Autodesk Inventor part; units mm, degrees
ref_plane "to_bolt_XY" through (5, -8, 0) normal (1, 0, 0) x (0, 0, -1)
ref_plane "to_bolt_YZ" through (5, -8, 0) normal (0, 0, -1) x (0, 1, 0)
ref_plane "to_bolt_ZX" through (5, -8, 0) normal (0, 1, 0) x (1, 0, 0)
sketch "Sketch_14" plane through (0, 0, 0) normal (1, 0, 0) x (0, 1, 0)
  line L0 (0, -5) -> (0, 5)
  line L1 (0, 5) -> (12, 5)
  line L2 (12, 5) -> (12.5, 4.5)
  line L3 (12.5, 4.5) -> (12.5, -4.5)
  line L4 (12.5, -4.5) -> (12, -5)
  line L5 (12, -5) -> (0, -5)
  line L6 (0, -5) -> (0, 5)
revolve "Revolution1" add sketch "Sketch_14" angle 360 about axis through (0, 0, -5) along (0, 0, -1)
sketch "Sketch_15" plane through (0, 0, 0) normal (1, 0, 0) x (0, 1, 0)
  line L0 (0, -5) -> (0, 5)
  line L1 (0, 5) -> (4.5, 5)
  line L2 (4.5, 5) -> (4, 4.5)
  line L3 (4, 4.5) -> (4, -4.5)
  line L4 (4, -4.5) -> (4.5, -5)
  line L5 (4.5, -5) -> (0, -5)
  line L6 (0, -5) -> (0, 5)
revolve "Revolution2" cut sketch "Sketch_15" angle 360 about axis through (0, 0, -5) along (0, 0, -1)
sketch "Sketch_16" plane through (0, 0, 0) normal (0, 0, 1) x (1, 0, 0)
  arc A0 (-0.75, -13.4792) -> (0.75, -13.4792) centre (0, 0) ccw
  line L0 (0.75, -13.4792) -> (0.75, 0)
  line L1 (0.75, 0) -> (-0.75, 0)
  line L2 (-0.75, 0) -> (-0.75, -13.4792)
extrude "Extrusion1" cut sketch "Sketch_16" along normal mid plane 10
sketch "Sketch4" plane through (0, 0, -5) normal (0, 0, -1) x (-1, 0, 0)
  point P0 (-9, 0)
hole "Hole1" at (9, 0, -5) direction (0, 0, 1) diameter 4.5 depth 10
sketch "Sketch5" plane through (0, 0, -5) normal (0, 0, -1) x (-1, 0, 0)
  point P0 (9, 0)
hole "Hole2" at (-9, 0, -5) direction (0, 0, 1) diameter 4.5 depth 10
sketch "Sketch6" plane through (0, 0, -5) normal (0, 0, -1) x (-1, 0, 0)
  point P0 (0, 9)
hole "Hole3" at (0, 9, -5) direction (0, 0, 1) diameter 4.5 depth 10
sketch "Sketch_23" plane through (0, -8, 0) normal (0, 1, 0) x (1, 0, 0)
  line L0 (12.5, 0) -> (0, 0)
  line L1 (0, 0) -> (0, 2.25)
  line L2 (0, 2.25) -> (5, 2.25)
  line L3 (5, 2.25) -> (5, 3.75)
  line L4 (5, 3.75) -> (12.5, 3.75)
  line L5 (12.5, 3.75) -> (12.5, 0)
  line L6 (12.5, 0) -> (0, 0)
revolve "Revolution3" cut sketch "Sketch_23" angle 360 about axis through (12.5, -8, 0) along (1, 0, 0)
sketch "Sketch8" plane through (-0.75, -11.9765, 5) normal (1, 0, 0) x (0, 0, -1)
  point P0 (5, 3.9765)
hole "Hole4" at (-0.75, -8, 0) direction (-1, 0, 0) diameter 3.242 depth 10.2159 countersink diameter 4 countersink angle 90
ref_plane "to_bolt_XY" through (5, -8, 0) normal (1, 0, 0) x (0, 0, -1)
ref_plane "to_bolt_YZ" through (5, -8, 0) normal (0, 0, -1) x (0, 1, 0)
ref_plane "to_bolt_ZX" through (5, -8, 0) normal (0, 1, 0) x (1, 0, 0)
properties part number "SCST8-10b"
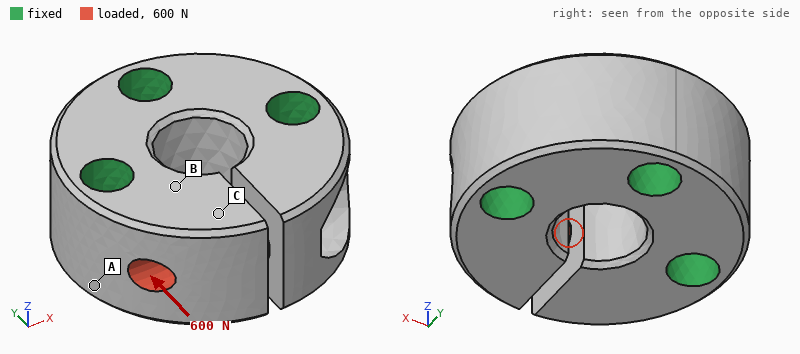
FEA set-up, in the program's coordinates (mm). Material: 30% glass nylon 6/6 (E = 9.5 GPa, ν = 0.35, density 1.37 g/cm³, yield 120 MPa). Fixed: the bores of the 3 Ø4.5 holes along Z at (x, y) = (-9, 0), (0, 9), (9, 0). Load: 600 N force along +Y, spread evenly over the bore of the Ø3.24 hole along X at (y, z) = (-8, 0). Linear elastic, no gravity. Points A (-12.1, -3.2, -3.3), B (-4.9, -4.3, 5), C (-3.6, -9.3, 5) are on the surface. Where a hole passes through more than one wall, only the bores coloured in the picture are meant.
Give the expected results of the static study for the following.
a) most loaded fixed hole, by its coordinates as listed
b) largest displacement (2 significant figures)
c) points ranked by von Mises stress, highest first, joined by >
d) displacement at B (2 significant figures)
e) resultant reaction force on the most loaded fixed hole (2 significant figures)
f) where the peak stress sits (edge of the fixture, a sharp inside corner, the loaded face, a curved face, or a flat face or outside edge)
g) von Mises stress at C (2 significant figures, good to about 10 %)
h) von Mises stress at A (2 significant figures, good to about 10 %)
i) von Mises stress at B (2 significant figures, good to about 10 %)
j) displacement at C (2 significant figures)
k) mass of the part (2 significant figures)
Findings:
(-9, 0)
35 µm
B > A > C
10.0 µm
530 N
the loaded face
2.5 MPa
6.5 MPa
10.0 MPa
21 µm
4.7 g
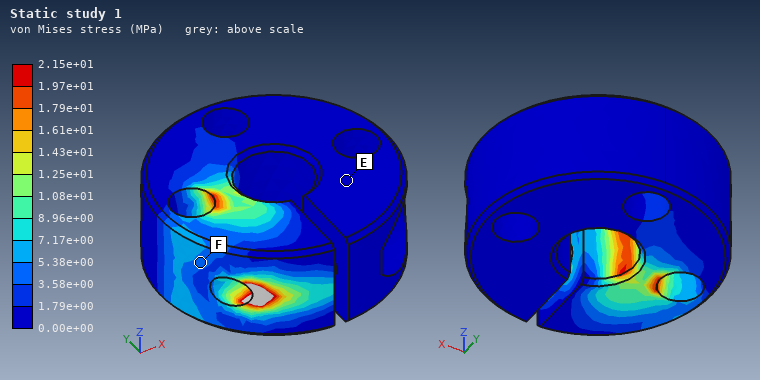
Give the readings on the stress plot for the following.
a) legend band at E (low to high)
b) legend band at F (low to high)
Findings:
0.00e+00 to 1.79e+00 MPa
3.58e+00 to 5.38e+00 MPa
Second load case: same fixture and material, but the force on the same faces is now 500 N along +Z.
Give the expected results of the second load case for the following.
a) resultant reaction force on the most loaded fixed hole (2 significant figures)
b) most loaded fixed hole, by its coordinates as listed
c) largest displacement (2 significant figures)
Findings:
510 N
(-9, 0)
45 µm
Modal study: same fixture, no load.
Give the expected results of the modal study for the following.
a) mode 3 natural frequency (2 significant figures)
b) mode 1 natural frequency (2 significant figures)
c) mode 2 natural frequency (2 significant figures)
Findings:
19 kHz
18 kHz
18 kHz
